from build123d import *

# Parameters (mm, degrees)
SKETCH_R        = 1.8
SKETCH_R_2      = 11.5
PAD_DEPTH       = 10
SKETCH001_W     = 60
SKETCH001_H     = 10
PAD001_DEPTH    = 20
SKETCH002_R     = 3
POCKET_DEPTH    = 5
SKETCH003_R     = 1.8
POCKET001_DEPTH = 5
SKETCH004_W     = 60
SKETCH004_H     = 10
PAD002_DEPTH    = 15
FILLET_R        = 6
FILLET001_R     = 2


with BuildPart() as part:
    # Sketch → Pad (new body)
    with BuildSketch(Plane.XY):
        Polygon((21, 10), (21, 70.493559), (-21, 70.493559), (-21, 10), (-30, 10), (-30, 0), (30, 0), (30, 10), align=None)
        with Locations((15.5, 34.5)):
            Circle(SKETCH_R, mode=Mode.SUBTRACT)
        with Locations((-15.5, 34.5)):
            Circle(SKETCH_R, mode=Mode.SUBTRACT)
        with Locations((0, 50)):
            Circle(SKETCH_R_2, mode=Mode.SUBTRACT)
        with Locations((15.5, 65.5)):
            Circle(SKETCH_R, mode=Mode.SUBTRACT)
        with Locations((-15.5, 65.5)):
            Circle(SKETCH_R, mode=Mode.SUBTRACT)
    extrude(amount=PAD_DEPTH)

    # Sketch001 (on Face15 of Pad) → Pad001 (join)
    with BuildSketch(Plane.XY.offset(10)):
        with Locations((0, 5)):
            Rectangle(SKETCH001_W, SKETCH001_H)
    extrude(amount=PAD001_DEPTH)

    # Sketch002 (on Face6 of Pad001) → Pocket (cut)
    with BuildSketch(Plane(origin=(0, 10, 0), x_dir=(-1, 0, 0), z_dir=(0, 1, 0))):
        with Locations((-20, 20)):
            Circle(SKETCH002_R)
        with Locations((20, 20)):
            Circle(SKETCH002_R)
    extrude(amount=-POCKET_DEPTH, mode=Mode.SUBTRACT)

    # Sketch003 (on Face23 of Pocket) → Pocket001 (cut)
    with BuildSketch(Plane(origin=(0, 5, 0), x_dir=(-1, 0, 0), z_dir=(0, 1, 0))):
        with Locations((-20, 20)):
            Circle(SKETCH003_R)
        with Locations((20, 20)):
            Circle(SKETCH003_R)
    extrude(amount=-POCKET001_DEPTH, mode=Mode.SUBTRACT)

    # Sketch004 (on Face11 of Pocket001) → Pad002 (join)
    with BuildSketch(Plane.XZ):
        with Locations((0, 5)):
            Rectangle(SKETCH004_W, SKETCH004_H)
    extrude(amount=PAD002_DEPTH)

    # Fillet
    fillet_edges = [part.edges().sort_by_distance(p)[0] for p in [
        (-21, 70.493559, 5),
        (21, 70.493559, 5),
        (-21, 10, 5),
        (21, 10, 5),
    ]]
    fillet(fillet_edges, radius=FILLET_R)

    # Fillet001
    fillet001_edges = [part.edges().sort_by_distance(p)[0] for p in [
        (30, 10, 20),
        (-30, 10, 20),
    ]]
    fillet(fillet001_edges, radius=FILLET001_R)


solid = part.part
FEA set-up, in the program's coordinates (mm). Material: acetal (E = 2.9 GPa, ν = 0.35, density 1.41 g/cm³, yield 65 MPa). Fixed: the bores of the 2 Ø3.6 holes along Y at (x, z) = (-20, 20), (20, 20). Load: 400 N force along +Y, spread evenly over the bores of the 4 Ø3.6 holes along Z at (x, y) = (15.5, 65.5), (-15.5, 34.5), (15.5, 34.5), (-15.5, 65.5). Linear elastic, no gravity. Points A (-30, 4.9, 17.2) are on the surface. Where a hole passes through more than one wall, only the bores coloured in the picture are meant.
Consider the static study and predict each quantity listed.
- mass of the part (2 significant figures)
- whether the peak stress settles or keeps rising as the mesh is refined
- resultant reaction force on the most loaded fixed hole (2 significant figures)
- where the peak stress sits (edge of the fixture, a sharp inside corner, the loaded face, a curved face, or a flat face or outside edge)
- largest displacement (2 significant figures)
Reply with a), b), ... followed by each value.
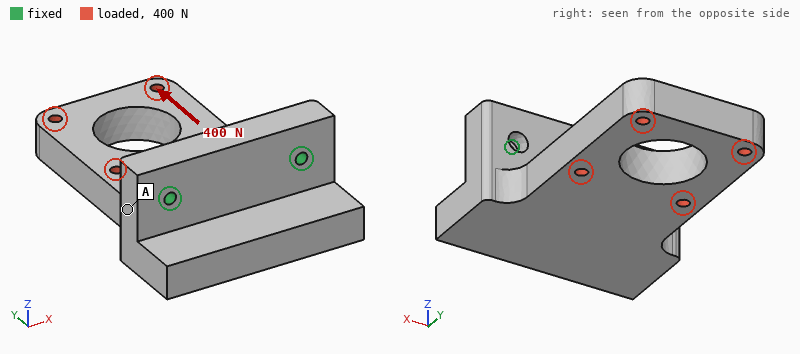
a) 67 g
b) keeps rising
c) 200 N
d) edge of the fixture
e) 1.1 mm
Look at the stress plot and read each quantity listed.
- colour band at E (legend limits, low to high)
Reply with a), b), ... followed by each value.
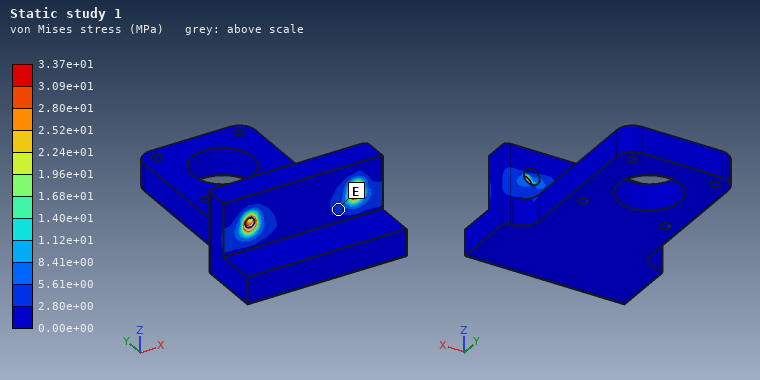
a) 2.80e+00 to 5.61e+00 MPa
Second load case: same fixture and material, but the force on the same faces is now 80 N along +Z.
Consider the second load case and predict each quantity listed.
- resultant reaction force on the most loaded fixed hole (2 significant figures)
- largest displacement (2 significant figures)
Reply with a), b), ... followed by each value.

a) 51 N
b) 1.2 mm
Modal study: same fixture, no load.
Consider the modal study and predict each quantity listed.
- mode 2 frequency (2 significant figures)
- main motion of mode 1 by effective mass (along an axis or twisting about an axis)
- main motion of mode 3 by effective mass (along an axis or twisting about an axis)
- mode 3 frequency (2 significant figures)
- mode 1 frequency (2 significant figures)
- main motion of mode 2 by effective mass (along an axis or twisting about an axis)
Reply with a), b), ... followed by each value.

a) 1100 Hz
b) along Z
c) along Y
d) 1300 Hz
e) 340 Hz
f) along X
